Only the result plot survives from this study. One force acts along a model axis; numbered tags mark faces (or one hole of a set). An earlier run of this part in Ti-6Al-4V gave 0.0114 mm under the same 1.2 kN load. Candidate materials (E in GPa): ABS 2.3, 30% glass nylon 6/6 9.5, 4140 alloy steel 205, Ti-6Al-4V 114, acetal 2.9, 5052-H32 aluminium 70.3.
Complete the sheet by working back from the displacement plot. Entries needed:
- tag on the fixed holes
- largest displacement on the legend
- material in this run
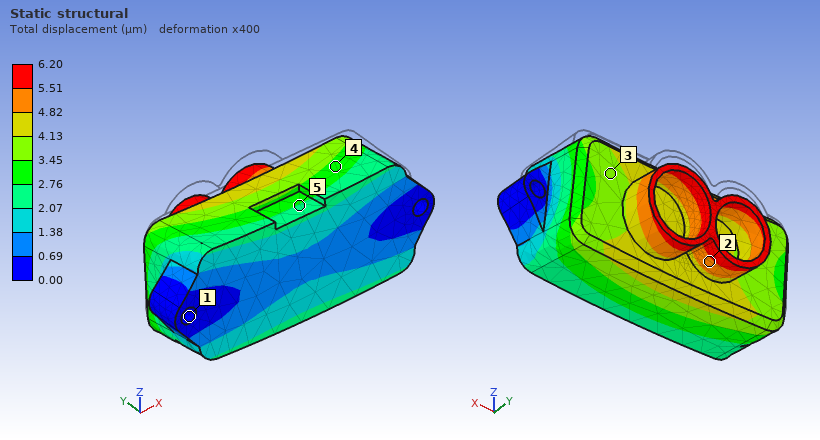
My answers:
1
6.20 µm
4140 alloy steel
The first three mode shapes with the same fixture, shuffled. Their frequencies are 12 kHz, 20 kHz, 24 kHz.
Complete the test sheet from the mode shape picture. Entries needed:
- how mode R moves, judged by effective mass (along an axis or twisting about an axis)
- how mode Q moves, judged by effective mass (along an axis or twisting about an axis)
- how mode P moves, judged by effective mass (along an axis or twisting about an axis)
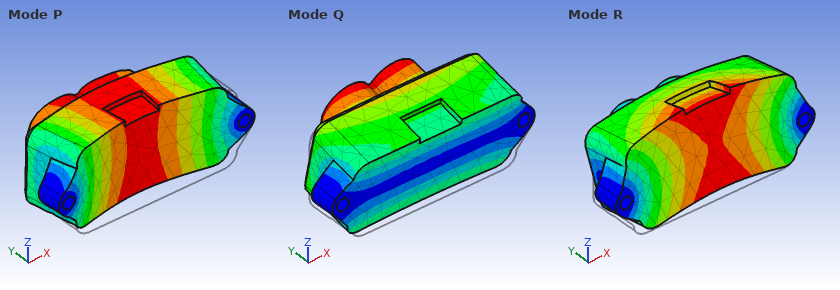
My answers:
along Z
along Z
along Y
